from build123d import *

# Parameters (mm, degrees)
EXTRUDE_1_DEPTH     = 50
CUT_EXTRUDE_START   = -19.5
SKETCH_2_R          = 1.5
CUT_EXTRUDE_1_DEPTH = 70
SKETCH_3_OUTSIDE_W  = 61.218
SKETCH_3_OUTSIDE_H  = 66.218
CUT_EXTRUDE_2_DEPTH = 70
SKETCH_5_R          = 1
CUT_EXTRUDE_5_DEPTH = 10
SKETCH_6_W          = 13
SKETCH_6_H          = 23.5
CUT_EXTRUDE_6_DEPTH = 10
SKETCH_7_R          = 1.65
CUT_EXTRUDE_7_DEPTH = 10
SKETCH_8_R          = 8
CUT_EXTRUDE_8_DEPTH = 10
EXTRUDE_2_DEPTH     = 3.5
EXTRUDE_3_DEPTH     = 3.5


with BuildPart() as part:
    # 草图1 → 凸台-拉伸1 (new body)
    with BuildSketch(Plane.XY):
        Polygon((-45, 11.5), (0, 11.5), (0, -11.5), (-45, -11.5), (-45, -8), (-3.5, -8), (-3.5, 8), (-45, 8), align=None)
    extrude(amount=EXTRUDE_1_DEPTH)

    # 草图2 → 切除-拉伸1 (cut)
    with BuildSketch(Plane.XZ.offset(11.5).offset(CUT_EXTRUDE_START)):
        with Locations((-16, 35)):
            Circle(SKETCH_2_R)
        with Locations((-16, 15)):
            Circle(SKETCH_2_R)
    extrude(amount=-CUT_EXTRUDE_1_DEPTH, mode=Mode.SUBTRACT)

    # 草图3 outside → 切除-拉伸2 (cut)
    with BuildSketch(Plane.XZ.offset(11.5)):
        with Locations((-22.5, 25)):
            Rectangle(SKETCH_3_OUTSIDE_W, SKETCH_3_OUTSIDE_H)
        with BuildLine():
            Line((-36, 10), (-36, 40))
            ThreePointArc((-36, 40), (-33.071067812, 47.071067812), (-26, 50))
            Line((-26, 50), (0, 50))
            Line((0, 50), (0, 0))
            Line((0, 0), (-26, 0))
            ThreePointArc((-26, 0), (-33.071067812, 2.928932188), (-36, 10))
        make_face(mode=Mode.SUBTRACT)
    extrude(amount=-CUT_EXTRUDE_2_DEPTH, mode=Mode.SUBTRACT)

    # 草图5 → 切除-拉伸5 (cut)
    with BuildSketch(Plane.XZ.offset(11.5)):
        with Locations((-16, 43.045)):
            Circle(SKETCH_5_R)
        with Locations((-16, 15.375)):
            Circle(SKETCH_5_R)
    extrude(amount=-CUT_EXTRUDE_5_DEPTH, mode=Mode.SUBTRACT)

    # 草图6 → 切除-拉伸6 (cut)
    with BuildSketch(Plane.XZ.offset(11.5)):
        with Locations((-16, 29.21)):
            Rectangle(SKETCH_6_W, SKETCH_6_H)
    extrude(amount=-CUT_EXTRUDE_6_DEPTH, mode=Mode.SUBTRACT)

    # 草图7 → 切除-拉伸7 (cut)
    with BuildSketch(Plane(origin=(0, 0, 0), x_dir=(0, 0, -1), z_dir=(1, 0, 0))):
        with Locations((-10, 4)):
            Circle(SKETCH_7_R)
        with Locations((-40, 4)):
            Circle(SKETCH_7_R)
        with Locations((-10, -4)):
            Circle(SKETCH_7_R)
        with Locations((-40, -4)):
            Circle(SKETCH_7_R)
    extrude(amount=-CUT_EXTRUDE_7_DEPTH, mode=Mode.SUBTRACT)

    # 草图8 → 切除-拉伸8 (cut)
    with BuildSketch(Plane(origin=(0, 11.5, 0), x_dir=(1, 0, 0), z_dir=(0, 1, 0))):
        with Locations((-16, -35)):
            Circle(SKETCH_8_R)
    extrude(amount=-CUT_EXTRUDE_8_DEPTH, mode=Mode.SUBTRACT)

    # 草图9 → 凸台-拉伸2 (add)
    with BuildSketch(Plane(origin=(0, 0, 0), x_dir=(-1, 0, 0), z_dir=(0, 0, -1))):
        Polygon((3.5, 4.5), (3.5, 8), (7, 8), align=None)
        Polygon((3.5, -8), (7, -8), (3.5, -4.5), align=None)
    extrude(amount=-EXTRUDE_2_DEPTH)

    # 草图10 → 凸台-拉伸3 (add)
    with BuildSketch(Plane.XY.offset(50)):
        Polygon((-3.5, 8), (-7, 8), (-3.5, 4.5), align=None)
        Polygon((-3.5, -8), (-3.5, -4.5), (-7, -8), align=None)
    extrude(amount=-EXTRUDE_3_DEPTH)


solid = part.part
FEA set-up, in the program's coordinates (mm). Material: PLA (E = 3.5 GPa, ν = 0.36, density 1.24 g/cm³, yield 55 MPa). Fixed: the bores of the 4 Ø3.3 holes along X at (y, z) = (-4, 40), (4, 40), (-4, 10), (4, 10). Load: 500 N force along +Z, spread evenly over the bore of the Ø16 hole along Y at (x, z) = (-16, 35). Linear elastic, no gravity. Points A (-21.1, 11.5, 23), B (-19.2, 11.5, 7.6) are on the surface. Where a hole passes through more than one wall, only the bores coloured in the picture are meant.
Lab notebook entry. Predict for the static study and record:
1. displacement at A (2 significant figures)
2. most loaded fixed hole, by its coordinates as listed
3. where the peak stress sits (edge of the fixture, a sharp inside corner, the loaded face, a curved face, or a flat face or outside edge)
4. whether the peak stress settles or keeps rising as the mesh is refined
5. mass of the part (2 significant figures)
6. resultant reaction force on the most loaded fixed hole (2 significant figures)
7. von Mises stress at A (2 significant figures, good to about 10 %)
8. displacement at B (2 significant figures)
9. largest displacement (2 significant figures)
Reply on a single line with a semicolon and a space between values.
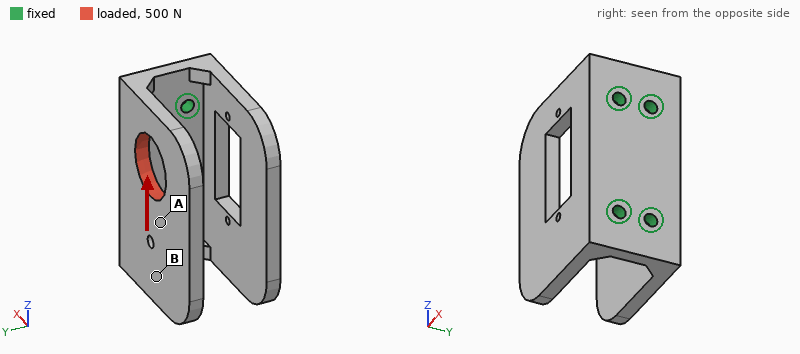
0.17 mm; (4, 40); edge of the fixture; keeps rising; 16 g; 350 N; 5.5 MPa; 0.21 mm; 0.36 mm
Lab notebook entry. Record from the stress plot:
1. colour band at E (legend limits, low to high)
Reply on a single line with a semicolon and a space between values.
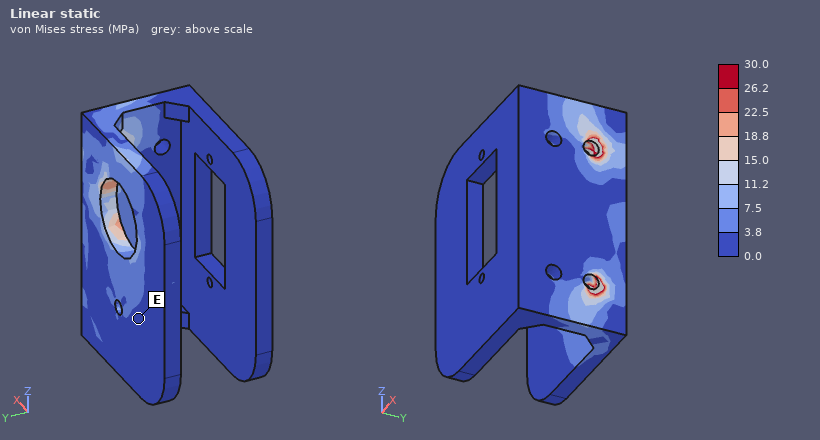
0.0 to 3.8 MPa
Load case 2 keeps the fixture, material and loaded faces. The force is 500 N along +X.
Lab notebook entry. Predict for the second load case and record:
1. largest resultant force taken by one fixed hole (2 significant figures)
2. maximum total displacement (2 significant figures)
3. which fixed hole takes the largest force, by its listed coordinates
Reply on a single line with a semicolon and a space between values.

460 N; 0.67 mm; (4, 40)
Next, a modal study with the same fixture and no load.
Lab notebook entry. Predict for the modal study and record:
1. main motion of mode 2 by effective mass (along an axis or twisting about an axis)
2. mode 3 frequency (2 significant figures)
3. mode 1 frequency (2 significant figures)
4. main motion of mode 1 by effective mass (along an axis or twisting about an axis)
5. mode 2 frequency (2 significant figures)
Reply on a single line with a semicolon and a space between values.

along Y; 1300 Hz; 600 Hz; along Y; 670 Hz
